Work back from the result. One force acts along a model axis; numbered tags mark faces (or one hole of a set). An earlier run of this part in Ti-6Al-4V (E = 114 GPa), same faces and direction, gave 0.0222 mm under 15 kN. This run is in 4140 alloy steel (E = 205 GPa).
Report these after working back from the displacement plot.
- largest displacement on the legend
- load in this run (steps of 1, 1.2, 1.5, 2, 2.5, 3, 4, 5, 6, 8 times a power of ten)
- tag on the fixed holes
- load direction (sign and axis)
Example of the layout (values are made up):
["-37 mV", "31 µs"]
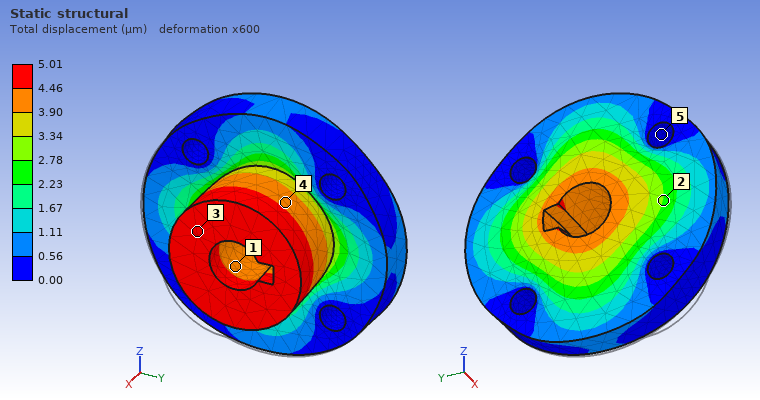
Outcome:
["5.01 µm", "6 kN", "5", "-X"]
